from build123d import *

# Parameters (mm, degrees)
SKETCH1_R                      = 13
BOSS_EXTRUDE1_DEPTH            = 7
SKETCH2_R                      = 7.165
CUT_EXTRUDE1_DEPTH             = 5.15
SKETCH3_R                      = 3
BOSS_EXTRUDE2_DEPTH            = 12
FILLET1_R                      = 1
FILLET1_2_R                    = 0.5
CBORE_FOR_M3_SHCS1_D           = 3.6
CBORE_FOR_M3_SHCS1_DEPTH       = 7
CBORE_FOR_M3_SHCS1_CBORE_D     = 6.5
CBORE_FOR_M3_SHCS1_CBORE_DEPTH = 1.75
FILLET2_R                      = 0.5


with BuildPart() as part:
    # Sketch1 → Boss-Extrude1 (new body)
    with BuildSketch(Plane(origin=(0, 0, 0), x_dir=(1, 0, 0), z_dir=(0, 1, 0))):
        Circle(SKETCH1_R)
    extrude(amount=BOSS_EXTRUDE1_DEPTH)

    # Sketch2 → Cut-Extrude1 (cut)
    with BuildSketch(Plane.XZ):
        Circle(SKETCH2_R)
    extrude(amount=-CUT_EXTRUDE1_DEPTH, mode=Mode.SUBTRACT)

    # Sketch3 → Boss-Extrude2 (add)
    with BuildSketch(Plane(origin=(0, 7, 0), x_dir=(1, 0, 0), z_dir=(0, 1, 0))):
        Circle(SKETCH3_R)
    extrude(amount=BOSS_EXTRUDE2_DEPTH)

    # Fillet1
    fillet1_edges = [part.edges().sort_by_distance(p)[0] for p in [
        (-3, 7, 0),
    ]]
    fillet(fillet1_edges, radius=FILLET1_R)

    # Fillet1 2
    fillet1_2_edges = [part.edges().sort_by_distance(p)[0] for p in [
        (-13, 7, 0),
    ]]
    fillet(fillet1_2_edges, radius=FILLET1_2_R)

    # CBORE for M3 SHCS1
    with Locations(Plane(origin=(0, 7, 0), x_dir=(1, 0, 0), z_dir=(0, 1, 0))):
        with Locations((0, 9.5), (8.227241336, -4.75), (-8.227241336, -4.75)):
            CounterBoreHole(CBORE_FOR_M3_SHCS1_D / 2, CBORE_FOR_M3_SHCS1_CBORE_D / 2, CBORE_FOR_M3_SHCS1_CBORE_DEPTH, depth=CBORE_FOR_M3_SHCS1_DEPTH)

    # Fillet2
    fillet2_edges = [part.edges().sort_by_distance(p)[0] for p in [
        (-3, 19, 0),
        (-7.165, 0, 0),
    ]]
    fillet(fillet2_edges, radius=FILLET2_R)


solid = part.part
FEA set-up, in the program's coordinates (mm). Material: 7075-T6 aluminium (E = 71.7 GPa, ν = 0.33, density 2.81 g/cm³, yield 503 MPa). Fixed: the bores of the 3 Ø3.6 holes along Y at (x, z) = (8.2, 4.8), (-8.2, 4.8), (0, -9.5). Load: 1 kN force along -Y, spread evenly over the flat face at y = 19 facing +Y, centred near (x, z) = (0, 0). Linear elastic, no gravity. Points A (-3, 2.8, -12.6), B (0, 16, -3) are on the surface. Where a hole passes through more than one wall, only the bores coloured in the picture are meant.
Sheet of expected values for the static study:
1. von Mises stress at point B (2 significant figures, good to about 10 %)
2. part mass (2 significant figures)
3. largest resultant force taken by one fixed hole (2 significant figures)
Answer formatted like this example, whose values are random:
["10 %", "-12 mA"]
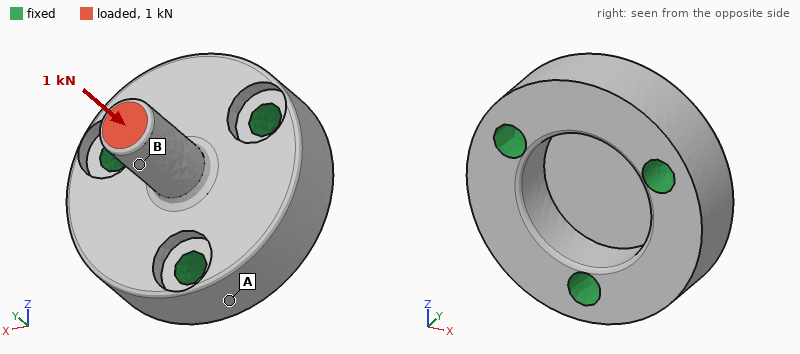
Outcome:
["34 MPa", "8.1 g", "390 N"]
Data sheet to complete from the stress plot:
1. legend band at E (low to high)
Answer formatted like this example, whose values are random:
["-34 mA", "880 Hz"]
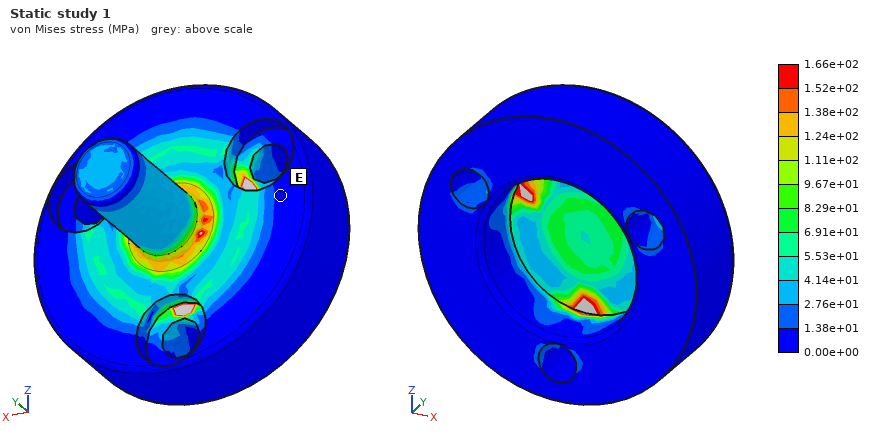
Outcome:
["0.00e+00 to 1.38e+01 MPa"]
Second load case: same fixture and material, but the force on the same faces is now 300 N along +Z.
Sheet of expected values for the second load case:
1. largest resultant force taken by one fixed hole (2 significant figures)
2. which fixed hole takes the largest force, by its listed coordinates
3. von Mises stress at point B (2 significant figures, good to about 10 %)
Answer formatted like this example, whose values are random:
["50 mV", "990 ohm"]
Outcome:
["330 N", "(0, -9.5)", "43 MPa"]
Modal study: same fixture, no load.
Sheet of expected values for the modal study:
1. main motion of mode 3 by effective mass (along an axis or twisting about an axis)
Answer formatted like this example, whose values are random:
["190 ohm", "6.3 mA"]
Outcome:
["along Y"]
